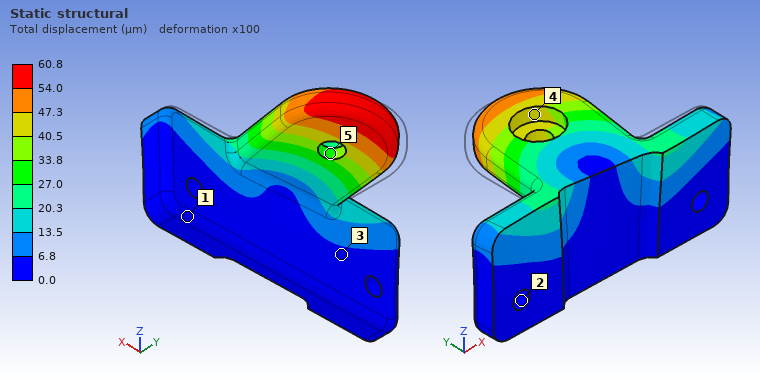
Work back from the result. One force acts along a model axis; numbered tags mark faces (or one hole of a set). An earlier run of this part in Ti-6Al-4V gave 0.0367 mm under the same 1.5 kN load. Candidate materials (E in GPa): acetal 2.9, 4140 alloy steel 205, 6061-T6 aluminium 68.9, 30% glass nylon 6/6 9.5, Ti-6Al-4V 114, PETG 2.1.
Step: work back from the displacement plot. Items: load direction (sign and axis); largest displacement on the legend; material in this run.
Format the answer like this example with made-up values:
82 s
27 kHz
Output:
+X
60.8 µm
6061-T6 aluminium
